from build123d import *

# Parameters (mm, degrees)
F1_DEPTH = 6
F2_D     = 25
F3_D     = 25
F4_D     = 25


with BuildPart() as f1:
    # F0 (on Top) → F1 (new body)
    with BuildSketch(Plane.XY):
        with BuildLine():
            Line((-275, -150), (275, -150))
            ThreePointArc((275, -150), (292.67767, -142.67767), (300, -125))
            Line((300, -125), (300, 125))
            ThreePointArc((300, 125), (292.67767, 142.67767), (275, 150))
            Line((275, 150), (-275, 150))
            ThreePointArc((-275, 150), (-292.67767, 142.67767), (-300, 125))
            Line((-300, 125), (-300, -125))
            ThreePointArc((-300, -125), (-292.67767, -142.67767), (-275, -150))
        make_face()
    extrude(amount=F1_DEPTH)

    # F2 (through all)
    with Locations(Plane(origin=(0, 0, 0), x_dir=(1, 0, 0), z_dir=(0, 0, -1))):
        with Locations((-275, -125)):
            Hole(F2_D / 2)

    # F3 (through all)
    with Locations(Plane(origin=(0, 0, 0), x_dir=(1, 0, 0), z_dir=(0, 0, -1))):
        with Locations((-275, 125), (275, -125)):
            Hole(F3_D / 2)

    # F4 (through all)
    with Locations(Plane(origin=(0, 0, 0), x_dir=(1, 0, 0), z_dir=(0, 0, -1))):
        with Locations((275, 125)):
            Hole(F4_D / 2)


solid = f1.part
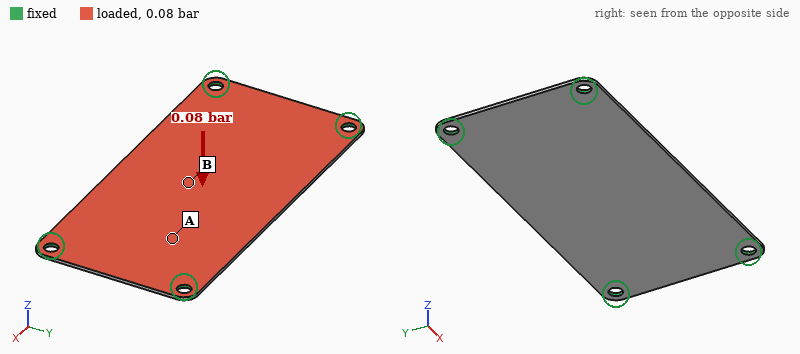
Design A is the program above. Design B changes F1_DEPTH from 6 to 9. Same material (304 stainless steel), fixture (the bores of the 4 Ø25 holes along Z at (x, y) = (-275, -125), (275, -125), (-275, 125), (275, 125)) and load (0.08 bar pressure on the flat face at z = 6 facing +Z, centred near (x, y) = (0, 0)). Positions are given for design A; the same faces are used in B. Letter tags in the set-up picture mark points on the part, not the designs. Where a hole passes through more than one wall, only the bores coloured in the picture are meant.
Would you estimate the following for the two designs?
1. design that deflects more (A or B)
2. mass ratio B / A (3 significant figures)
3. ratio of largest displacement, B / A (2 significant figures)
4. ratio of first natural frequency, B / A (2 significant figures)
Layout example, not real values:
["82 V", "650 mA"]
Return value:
["A", "1.50", "0.30", "1.5"]
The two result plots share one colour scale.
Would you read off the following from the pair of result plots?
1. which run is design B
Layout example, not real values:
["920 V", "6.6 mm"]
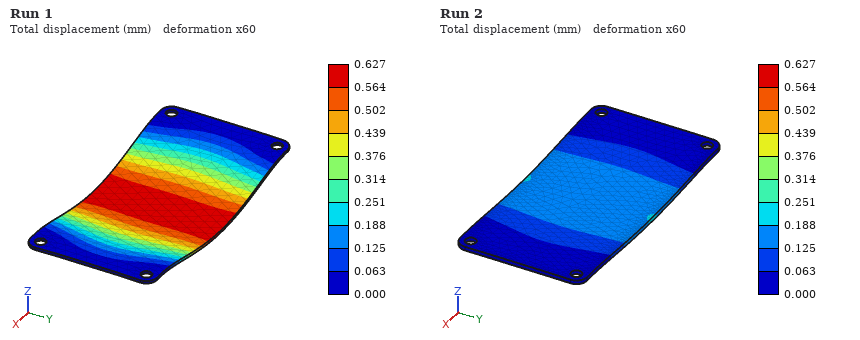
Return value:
["Run 2"]
